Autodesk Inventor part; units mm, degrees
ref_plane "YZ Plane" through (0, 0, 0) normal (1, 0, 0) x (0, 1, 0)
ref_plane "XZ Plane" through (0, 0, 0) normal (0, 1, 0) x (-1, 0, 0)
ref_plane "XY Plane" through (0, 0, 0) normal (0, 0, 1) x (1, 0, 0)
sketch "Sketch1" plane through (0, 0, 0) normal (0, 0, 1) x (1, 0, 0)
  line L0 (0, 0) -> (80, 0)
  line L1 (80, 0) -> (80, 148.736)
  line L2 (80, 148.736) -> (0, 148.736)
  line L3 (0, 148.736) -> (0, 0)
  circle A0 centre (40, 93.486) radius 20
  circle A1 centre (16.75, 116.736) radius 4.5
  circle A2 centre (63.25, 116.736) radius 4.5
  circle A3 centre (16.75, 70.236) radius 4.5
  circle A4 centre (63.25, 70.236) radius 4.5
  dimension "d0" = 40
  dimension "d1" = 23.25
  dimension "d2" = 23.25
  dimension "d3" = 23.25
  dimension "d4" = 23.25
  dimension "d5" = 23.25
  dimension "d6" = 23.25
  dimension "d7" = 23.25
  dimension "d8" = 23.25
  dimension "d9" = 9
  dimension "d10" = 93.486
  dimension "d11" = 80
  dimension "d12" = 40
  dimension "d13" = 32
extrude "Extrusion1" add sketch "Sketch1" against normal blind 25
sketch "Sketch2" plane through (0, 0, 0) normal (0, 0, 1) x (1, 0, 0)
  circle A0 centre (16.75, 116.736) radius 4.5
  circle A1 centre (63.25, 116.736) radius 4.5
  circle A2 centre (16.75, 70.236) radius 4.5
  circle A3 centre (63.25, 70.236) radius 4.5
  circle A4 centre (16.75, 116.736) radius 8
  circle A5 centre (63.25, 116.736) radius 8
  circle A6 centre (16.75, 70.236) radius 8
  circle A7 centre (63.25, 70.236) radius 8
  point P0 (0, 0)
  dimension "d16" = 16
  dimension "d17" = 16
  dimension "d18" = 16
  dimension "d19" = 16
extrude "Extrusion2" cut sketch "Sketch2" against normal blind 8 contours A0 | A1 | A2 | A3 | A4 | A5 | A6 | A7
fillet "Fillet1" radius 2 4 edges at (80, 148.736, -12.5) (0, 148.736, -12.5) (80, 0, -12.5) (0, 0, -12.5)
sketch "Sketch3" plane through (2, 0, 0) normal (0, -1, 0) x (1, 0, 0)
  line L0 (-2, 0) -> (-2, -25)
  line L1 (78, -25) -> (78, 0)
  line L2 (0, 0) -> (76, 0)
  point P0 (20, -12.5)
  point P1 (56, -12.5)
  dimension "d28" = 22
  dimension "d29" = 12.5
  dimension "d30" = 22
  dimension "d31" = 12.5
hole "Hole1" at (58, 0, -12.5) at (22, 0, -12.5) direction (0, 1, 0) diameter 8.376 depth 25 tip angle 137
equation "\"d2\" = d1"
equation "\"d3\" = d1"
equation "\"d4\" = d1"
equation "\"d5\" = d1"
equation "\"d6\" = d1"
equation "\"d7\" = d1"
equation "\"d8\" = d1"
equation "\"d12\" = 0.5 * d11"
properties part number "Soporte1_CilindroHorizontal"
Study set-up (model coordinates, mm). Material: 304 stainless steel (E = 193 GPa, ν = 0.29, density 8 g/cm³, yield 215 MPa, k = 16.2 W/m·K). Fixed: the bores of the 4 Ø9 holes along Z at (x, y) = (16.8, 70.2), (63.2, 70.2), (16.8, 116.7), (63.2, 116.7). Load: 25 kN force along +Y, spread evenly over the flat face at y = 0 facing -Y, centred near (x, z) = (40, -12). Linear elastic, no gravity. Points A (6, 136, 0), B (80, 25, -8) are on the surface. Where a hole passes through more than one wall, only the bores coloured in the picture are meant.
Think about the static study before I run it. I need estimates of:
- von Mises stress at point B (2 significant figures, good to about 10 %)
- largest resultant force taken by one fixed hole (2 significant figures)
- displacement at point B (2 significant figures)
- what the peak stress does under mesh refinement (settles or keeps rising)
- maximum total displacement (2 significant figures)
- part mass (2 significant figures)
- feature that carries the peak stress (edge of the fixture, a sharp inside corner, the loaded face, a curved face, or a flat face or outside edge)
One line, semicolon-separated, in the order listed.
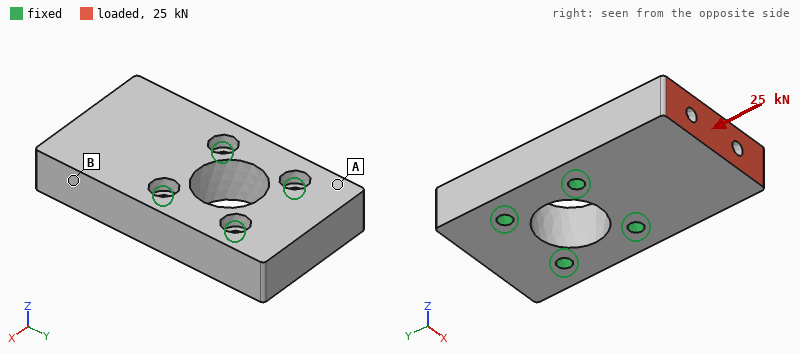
12 MPa; 11 kN; 6.3 µm; keeps rising; 10 µm; 2.0 kg; edge of the fixture
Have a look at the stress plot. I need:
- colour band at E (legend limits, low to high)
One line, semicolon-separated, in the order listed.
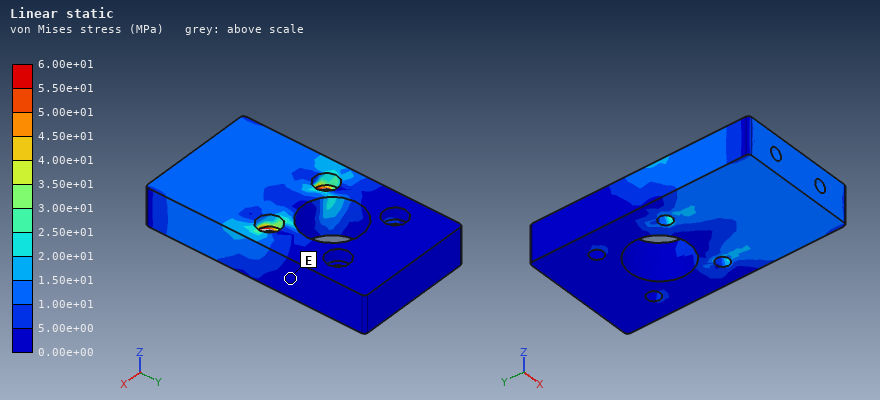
0.00e+00 to 5.00e+00 MPa
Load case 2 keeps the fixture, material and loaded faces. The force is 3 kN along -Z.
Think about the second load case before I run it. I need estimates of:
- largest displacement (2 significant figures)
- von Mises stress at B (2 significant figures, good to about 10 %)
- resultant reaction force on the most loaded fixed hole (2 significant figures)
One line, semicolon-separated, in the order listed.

31 µm; 6.1 MPa; 2.4 kN
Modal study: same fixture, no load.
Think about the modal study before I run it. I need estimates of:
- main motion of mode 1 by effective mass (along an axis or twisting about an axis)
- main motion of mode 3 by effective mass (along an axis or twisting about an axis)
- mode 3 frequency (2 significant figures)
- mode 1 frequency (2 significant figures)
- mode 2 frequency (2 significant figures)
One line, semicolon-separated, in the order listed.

along Z; along X; 6900 Hz; 2800 Hz; 6300 Hz
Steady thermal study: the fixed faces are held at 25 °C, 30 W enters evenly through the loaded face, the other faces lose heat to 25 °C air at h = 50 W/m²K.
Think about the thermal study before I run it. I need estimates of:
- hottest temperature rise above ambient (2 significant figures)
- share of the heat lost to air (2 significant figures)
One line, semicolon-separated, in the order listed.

46 K; 58 %
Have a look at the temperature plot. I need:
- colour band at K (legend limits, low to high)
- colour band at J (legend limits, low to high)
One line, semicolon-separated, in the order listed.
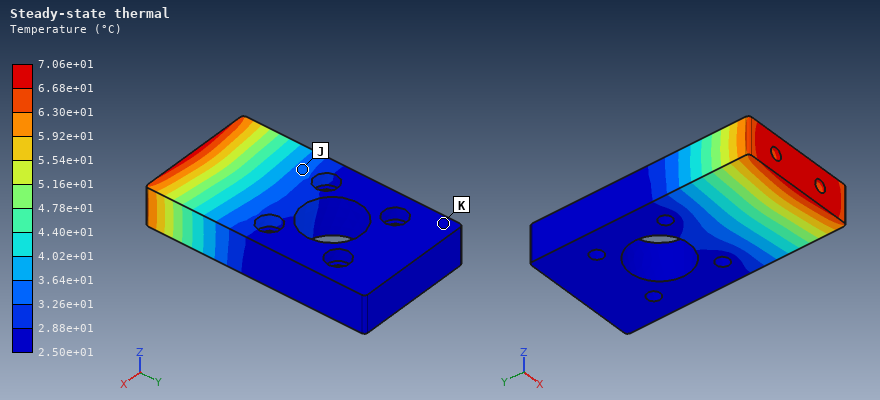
2.50e+01 to 2.88e+01 °C; 3.26e+01 to 3.64e+01 °C
